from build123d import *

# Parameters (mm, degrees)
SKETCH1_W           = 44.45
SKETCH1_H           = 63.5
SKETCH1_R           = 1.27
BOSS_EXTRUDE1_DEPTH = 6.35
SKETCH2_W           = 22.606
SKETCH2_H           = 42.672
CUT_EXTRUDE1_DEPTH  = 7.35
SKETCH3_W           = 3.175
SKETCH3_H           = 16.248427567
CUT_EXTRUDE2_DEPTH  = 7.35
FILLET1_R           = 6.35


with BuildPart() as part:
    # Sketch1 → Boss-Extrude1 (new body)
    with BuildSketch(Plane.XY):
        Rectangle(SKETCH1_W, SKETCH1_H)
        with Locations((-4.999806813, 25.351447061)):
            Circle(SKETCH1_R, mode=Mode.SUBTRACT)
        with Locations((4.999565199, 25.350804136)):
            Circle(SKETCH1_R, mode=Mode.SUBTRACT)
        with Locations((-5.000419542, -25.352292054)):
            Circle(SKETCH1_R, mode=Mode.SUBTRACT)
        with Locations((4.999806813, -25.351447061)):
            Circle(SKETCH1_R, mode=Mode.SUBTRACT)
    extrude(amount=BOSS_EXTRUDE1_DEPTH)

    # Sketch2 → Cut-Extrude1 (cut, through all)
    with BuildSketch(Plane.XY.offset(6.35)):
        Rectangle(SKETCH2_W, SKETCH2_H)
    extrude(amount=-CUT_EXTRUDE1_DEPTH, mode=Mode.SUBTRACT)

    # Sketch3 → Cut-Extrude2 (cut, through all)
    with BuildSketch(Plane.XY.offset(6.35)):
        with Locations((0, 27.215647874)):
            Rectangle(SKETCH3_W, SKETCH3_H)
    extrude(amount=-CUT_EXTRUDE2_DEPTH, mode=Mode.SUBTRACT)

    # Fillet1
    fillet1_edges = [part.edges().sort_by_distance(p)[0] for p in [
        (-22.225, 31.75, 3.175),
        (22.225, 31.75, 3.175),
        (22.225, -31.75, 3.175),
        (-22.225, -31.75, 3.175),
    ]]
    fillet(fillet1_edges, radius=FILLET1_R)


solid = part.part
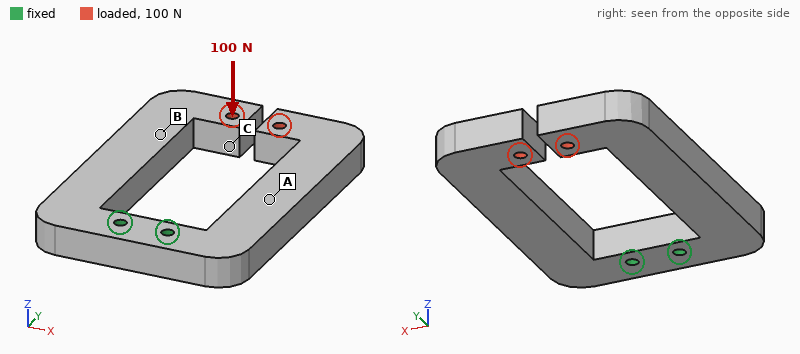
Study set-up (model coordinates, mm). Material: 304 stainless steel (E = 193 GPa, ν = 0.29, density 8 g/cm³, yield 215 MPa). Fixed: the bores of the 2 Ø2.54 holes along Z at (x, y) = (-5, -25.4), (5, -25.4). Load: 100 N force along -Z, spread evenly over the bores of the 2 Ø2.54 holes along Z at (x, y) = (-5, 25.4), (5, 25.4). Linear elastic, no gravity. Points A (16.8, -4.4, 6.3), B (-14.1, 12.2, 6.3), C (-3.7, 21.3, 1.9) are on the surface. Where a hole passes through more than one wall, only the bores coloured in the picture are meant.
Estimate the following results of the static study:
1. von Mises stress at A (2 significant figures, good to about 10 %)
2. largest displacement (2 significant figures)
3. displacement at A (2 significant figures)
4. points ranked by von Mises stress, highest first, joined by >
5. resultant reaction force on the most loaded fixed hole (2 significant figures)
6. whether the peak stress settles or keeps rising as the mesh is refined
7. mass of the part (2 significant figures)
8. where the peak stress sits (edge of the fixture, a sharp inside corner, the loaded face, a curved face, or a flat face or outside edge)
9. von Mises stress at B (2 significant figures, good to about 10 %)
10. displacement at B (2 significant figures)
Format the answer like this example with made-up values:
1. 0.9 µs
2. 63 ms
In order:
1. 22 MPa
2. 99 µm
3. 22 µm
4. A > B > C
5. 50 N
6. keeps rising
7. 90 g
8. edge of the fixture
9. 12 MPa
10. 52 µm
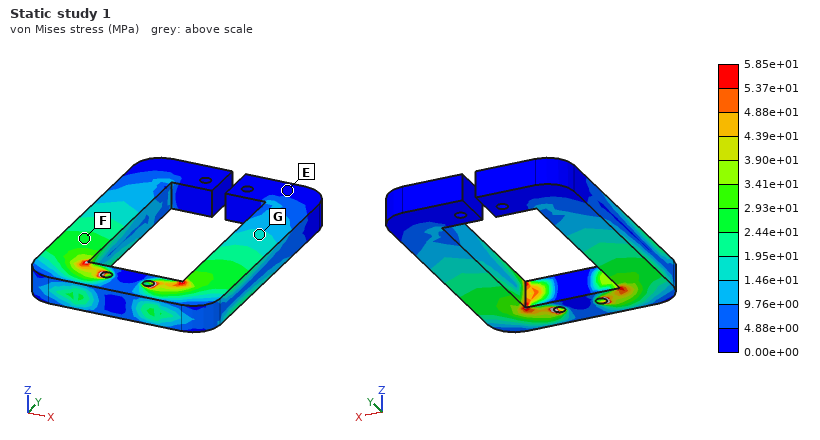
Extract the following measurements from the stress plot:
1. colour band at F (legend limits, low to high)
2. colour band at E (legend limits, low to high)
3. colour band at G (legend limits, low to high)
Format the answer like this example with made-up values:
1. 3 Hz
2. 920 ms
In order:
1. 2.44e+01 to 2.93e+01 MPa
2. 0.00e+00 to 4.88e+00 MPa
3. 1.46e+01 to 1.95e+01 MPa
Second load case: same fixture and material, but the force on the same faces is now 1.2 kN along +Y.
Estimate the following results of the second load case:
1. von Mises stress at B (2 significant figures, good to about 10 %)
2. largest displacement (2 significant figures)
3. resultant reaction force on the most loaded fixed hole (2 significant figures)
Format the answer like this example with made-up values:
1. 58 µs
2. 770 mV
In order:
1. 36 MPa
2. 0.11 mm
3. 600 N
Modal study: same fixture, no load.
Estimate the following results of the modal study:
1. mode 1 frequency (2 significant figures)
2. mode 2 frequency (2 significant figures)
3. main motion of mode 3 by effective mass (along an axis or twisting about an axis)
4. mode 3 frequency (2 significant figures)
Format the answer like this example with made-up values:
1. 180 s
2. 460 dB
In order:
1. 1000 Hz
2. 1000 Hz
3. along X
4. 1500 Hz
